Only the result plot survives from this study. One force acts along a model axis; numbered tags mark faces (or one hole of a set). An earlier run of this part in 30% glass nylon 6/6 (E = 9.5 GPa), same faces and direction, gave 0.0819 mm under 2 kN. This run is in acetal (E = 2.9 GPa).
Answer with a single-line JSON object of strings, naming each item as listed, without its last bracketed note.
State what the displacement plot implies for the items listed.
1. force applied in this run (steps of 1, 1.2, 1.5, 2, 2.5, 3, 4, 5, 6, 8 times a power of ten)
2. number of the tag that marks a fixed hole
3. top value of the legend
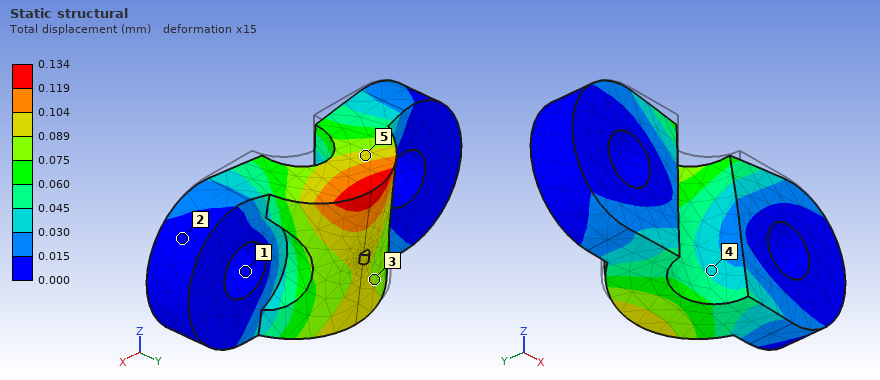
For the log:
{"force applied in this run": "1 kN", "number of the tag that marks a fixed hole": "1", "top value of the legend": "0.134 mm"}
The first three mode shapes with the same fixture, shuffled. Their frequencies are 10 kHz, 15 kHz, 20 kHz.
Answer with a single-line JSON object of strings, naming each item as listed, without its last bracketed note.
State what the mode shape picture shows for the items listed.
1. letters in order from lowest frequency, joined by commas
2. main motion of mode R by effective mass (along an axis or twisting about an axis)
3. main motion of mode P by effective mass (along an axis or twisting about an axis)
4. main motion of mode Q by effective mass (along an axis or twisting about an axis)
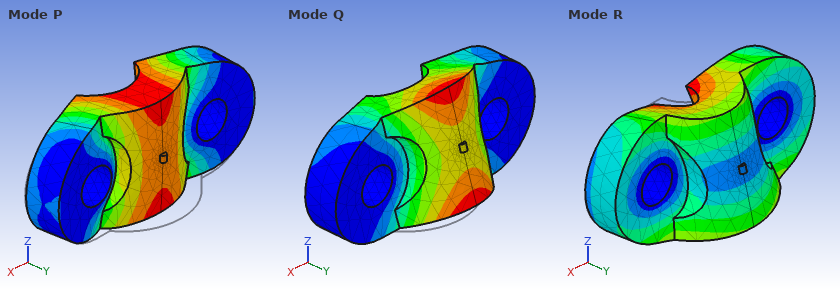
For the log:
{"letters in order from lowest frequency, joined by commas": "Q, P, R", "main motion of mode R by effective mass": "along Z", "main motion of mode P by effective mass": "along Y", "main motion of mode Q by effective mass": "along Z"}
